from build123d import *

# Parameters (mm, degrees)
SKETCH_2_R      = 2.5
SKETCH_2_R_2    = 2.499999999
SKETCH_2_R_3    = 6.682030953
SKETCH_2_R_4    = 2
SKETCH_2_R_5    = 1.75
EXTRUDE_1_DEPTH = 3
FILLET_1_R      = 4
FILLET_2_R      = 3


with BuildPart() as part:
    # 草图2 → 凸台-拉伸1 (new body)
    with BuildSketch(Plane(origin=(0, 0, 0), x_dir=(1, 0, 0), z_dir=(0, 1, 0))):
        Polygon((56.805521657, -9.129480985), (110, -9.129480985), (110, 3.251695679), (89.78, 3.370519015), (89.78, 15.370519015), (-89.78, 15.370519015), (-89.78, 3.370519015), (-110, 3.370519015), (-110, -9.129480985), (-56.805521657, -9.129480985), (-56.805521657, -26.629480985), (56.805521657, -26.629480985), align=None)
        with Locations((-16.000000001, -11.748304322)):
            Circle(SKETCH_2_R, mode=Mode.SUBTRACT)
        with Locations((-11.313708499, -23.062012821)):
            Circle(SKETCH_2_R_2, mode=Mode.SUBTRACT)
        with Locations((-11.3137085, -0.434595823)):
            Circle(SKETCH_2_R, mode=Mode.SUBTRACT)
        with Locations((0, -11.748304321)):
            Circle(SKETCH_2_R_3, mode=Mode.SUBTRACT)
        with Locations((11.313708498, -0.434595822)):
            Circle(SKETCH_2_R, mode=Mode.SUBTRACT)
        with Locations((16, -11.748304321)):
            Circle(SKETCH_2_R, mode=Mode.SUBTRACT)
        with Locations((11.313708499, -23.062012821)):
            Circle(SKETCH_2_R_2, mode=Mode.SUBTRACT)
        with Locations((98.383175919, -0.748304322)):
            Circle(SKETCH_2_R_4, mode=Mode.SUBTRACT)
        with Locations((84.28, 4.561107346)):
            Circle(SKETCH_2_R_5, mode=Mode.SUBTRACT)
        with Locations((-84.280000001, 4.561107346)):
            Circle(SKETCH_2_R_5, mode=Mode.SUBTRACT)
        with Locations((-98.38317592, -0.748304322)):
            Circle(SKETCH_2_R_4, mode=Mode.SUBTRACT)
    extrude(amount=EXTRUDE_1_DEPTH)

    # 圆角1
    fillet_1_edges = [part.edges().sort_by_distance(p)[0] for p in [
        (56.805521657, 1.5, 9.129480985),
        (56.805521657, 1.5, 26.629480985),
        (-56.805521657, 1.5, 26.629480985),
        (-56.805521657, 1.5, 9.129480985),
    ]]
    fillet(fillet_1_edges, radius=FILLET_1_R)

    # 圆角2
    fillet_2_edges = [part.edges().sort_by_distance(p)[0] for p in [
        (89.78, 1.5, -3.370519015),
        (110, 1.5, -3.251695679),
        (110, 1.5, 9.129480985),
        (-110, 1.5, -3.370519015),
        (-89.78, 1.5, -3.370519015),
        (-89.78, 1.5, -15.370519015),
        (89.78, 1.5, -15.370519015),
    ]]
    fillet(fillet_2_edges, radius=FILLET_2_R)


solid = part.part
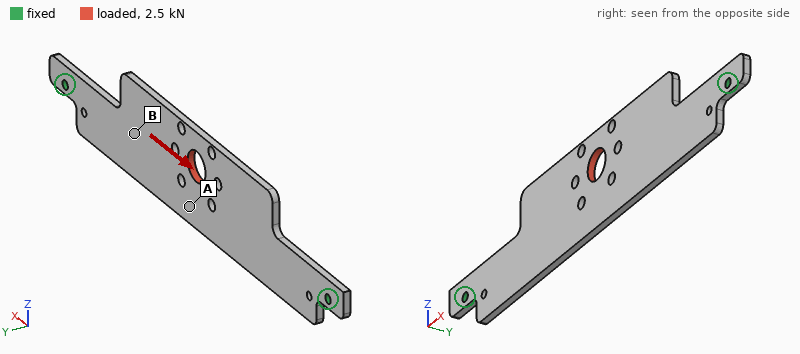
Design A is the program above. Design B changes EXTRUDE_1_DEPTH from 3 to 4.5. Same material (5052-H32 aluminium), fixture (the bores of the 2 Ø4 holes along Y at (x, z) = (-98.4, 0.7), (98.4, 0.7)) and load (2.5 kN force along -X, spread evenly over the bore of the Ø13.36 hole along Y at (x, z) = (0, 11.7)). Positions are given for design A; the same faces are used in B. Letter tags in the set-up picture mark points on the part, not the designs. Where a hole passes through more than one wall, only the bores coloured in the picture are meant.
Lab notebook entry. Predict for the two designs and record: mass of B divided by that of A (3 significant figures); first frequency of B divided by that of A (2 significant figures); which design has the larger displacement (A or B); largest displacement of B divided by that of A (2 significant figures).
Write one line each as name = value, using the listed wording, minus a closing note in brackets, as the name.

mass of B divided by that of A = 1.50
first frequency of B divided by that of A = 1.5
which design has the larger displacement = A
largest displacement of B divided by that of A = 0.67
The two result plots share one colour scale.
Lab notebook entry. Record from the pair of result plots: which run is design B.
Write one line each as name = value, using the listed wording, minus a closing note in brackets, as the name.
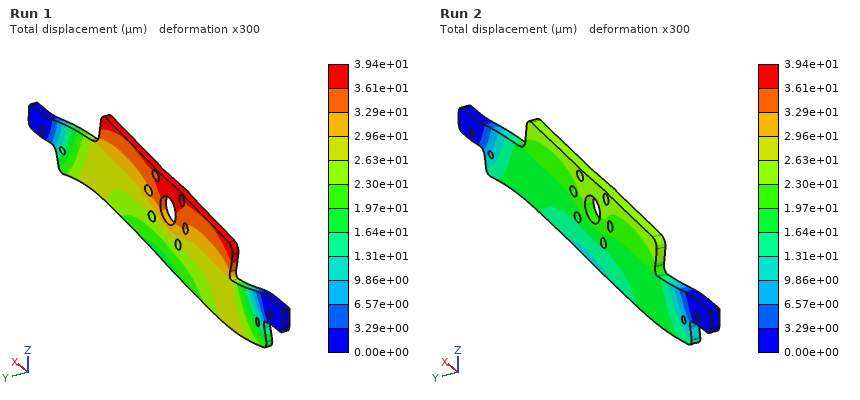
which run is design B = Run 2
